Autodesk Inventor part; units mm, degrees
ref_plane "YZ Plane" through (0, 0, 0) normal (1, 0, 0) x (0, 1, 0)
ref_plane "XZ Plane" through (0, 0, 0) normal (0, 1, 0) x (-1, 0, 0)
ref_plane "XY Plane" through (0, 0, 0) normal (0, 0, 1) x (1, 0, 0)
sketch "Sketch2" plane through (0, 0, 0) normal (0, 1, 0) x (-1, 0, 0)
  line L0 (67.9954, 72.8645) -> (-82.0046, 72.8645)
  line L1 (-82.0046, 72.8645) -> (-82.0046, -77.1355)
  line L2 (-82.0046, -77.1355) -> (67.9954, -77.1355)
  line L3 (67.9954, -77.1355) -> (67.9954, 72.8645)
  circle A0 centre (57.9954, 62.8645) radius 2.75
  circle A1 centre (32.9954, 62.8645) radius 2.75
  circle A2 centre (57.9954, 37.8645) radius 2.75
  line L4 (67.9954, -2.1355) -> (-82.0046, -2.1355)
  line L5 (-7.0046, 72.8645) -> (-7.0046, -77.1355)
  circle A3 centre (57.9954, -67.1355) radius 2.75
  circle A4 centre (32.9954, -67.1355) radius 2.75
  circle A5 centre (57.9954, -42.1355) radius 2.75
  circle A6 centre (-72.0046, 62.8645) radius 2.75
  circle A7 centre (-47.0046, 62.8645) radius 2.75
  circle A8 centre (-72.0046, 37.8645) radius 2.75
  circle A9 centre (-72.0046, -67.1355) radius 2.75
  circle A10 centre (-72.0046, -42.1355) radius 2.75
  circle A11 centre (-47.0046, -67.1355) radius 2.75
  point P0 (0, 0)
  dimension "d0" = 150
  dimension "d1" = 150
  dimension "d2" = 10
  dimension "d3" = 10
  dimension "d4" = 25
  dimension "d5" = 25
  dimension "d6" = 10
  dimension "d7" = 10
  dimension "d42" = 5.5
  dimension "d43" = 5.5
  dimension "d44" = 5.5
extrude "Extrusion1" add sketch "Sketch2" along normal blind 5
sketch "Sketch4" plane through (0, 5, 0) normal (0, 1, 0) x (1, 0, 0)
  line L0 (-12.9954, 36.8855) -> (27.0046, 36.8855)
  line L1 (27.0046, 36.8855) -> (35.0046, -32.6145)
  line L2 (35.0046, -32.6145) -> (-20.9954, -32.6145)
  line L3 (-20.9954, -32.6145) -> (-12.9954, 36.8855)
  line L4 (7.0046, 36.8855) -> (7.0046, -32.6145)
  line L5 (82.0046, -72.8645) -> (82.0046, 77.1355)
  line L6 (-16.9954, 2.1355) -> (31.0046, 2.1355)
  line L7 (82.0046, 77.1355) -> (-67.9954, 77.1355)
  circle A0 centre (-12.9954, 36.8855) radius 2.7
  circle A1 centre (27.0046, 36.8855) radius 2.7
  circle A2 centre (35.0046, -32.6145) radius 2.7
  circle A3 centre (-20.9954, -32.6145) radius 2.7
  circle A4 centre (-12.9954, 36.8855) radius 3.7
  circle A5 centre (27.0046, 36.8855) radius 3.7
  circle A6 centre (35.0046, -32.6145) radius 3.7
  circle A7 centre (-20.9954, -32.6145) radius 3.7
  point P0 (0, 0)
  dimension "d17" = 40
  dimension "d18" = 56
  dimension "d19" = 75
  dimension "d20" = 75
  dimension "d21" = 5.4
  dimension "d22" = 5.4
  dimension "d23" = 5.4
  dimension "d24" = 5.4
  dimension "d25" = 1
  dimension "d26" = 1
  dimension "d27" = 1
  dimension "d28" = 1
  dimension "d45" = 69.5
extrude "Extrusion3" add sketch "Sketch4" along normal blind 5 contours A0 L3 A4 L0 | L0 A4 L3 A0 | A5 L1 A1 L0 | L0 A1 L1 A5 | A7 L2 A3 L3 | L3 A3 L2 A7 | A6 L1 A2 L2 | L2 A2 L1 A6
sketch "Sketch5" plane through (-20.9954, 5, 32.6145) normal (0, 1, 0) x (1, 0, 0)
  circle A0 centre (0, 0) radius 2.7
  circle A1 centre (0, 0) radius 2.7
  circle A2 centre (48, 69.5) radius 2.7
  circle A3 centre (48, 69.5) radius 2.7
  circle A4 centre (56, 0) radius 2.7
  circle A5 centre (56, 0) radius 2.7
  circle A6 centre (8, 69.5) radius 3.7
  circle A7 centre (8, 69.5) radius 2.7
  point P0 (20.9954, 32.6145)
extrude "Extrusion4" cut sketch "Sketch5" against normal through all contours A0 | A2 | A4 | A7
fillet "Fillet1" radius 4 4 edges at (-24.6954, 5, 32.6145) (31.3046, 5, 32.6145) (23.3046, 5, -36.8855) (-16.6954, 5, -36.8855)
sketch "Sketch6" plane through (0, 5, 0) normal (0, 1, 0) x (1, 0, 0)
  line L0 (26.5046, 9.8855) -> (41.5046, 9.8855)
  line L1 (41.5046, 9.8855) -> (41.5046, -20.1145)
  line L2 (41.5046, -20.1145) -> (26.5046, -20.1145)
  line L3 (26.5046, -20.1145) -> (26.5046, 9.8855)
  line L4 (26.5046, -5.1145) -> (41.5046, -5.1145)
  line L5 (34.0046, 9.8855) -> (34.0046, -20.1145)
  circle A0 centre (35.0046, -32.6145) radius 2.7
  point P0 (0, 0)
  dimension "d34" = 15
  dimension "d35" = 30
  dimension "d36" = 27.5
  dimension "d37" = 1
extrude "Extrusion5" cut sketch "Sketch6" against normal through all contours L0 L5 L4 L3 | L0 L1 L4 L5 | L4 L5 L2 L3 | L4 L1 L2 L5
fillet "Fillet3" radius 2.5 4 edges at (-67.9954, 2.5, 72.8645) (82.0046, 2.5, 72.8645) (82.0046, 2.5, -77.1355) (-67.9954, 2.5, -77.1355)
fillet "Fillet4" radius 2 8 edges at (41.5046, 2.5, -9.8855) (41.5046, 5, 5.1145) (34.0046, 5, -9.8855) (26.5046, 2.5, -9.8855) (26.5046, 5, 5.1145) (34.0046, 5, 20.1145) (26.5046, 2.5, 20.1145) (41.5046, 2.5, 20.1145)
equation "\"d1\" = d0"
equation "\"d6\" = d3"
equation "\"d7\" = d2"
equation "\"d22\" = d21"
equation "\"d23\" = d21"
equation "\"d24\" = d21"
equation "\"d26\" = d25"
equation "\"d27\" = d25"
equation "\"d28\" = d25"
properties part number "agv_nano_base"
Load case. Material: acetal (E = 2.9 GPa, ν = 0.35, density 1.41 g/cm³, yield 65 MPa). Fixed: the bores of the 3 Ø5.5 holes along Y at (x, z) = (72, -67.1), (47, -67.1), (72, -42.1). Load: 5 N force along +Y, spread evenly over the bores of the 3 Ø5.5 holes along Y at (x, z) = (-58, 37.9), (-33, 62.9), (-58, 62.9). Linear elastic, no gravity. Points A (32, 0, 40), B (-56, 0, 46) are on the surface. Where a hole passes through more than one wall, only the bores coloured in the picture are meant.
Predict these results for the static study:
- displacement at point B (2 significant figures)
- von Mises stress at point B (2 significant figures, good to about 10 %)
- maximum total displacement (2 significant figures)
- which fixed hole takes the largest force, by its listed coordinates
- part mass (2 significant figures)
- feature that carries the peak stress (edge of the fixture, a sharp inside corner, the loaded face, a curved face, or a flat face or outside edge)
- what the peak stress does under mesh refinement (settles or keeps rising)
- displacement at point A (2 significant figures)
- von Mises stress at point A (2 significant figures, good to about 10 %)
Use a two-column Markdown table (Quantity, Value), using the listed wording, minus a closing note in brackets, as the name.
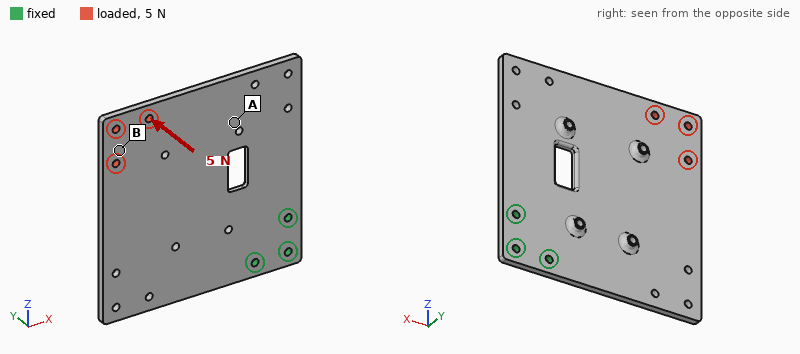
| Quantity | Value |
|---|---|
| displacement at point B | 2.0 mm |
| von Mises stress at point B | 0.28 MPa |
| maximum total displacement | 2.5 mm |
| which fixed hole takes the largest force, by its listed coordinates | (72, -67.1) |
| part mass | 150 g |
| feature that carries the peak stress | edge of the fixture |
| what the peak stress does under mesh refinement | keeps rising |
| displacement at point A | 0.82 mm |
| von Mises stress at point A | 0.54 MPa |
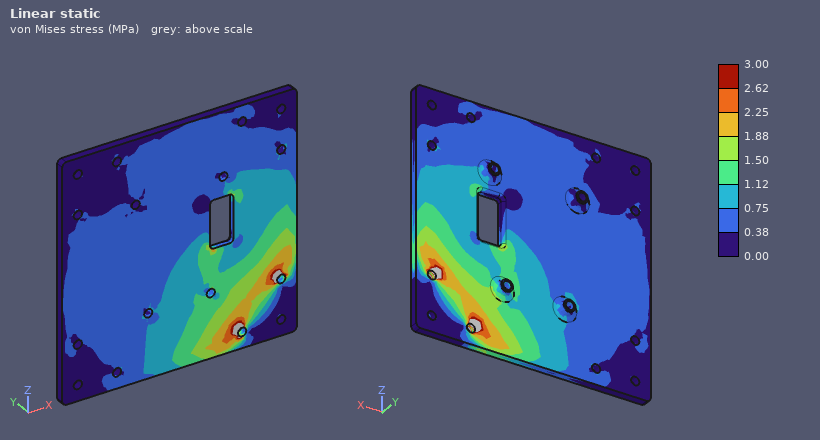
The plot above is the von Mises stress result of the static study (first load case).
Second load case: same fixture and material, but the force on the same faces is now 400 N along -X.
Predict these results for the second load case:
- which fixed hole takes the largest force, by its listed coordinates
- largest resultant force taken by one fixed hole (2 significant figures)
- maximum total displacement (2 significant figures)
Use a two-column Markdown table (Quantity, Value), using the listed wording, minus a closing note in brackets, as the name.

| Quantity | Value |
|---|---|
| which fixed hole takes the largest force, by its listed coordinates | (72, -42.1) |
| largest resultant force taken by one fixed hole | 1.2 kN |
| maximum total displacement | 1.2 mm |
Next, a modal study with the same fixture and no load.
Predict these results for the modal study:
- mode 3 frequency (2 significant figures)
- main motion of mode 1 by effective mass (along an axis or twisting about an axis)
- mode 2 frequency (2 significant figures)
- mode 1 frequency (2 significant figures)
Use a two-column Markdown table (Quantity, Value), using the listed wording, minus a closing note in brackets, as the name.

| Quantity | Value |
|---|---|
| mode 3 frequency | 190 Hz |
| main motion of mode 1 by effective mass | along Y |
| mode 2 frequency | 90 Hz |
| mode 1 frequency | 42 Hz |
